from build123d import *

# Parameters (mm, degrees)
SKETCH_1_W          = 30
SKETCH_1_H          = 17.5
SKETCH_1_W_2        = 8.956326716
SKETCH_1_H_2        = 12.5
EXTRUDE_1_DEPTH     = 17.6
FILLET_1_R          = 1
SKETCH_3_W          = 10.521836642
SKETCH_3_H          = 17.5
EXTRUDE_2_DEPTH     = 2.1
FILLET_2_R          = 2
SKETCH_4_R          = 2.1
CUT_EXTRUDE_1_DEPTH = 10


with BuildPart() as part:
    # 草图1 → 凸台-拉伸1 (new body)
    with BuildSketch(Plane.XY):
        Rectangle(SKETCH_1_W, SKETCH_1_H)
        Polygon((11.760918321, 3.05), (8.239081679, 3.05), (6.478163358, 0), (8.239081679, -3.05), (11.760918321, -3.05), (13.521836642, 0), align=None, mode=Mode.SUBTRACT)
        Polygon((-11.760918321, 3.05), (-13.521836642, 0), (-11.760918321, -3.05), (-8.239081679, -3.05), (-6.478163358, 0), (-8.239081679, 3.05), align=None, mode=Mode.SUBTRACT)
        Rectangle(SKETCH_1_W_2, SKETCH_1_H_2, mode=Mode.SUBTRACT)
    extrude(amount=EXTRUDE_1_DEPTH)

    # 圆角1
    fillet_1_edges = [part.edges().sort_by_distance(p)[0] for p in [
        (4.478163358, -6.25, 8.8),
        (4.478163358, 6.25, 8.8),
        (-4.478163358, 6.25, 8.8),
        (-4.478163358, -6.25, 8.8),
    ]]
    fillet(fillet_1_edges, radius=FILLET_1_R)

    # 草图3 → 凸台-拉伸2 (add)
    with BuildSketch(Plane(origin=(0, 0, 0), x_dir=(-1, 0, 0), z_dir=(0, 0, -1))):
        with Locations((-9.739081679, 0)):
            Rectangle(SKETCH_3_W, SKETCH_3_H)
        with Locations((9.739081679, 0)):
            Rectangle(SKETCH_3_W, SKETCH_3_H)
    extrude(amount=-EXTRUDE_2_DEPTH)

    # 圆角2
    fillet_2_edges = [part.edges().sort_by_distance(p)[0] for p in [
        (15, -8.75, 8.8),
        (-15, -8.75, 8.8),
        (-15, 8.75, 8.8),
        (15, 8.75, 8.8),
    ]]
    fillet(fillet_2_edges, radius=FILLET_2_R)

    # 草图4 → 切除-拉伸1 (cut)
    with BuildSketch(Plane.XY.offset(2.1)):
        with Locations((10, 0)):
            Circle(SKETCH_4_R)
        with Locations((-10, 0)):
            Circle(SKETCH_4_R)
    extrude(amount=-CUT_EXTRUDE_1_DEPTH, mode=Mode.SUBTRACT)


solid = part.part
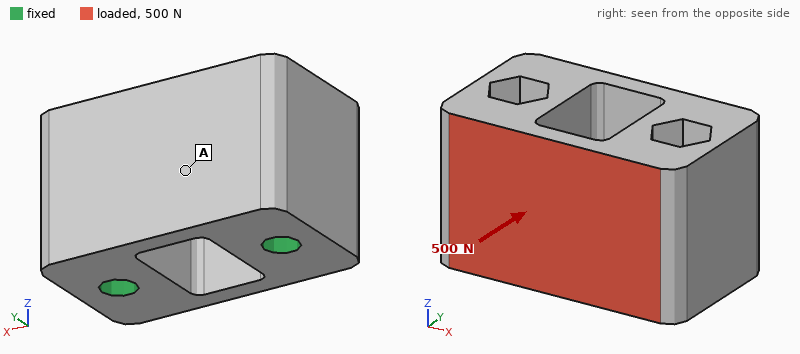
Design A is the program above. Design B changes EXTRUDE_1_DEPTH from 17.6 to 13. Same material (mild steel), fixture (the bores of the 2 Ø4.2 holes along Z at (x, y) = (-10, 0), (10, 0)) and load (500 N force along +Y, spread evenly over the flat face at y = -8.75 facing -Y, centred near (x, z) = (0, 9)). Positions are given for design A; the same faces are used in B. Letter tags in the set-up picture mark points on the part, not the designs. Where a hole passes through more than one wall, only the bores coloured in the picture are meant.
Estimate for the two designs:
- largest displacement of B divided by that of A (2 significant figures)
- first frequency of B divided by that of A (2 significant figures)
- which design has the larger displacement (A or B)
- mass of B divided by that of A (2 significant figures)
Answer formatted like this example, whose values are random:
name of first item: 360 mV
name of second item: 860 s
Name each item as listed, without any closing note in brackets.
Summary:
largest displacement of B divided by that of A: 0.62
first frequency of B divided by that of A: 1.4
which design has the larger displacement: A
mass of B divided by that of A: 0.74
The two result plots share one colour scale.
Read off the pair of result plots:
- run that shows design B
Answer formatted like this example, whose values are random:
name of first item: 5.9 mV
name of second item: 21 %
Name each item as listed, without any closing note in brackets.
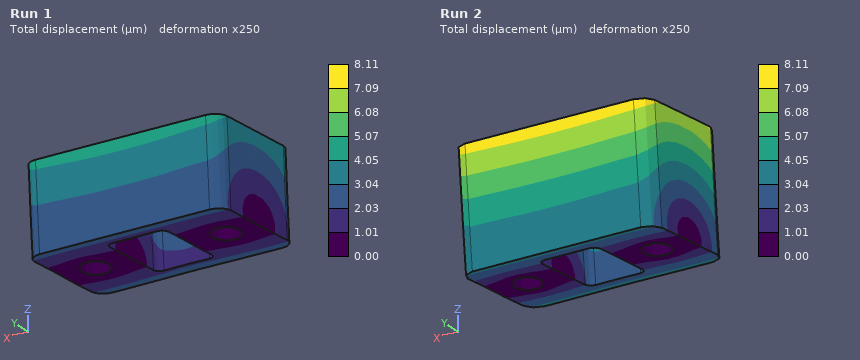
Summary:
run that shows design B: Run 1
